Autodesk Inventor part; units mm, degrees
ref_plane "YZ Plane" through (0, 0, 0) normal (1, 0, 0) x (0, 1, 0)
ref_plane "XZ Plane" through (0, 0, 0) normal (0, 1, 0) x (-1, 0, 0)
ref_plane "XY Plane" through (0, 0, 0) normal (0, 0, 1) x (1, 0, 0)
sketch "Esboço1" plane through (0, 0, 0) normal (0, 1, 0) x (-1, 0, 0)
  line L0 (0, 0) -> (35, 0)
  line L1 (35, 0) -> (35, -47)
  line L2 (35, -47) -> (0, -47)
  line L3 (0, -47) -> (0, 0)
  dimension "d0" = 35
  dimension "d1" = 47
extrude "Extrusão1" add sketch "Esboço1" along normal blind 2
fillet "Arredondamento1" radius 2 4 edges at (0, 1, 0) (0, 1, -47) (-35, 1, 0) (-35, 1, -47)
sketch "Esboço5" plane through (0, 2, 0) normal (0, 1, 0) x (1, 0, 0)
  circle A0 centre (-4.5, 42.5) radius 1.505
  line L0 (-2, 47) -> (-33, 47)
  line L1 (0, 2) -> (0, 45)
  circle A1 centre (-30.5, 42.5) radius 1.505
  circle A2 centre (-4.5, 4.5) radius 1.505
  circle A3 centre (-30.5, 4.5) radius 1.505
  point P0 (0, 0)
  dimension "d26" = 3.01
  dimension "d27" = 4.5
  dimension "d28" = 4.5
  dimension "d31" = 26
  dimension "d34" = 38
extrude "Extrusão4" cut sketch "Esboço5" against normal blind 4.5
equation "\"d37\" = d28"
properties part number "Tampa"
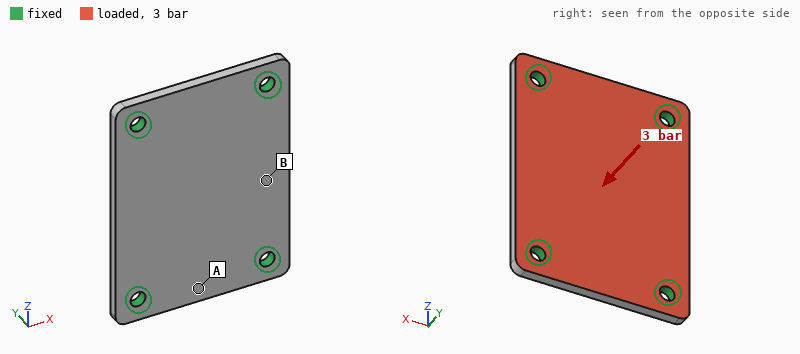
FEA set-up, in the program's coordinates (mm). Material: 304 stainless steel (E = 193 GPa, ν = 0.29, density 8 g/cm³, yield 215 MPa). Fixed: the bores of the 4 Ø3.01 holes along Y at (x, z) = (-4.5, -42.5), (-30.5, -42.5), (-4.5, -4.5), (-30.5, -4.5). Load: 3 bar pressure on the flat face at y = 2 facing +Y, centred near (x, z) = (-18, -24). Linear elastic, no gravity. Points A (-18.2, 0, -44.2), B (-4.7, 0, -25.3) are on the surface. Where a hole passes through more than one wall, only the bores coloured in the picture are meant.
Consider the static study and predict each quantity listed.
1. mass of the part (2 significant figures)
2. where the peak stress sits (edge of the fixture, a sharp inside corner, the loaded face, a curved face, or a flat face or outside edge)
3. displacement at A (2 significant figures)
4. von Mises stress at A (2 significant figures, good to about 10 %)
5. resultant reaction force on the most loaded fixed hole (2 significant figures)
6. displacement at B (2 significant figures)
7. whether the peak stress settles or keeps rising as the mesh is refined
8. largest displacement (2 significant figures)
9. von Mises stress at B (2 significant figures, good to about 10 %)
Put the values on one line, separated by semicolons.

26 g; edge of the fixture; 2.5 µm; 14 MPa; 120 N; 14 µm; keeps rising; 16 µm; 28 MPa
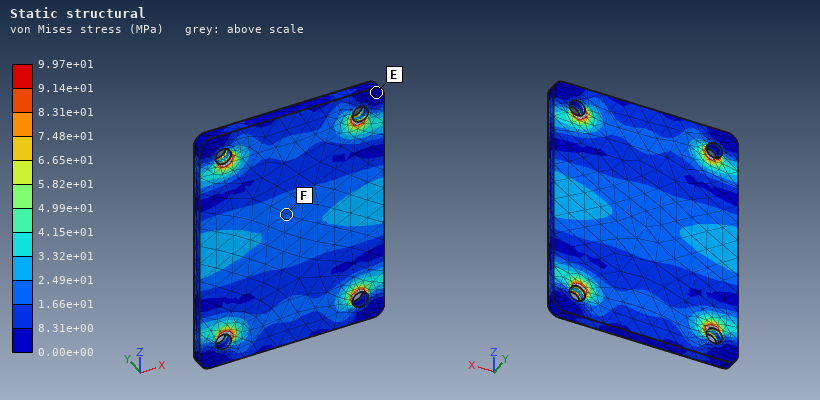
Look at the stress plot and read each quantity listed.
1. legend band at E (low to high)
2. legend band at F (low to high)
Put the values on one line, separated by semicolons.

0.00e+00 to 8.31e+00 MPa; 1.66e+01 to 2.49e+01 MPa
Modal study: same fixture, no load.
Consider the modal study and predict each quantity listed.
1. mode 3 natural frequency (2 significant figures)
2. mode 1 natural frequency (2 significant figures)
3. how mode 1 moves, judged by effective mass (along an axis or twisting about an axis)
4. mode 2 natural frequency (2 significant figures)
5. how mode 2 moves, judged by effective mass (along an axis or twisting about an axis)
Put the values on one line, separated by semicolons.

13 kHz; 6300 Hz; along Y; 8900 Hz; twisting about Z
